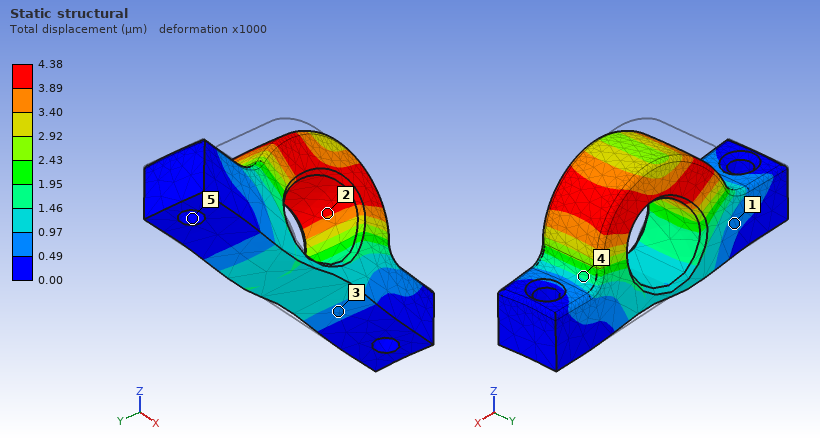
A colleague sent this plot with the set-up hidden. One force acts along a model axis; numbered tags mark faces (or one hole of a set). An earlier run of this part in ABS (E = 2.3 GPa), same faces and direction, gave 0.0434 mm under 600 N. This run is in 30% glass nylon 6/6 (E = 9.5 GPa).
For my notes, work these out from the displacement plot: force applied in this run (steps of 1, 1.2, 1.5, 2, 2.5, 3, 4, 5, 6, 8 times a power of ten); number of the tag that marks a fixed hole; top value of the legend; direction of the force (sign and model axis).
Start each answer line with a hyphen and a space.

- 250 N
- 5
- 4.38 µm
- +X
